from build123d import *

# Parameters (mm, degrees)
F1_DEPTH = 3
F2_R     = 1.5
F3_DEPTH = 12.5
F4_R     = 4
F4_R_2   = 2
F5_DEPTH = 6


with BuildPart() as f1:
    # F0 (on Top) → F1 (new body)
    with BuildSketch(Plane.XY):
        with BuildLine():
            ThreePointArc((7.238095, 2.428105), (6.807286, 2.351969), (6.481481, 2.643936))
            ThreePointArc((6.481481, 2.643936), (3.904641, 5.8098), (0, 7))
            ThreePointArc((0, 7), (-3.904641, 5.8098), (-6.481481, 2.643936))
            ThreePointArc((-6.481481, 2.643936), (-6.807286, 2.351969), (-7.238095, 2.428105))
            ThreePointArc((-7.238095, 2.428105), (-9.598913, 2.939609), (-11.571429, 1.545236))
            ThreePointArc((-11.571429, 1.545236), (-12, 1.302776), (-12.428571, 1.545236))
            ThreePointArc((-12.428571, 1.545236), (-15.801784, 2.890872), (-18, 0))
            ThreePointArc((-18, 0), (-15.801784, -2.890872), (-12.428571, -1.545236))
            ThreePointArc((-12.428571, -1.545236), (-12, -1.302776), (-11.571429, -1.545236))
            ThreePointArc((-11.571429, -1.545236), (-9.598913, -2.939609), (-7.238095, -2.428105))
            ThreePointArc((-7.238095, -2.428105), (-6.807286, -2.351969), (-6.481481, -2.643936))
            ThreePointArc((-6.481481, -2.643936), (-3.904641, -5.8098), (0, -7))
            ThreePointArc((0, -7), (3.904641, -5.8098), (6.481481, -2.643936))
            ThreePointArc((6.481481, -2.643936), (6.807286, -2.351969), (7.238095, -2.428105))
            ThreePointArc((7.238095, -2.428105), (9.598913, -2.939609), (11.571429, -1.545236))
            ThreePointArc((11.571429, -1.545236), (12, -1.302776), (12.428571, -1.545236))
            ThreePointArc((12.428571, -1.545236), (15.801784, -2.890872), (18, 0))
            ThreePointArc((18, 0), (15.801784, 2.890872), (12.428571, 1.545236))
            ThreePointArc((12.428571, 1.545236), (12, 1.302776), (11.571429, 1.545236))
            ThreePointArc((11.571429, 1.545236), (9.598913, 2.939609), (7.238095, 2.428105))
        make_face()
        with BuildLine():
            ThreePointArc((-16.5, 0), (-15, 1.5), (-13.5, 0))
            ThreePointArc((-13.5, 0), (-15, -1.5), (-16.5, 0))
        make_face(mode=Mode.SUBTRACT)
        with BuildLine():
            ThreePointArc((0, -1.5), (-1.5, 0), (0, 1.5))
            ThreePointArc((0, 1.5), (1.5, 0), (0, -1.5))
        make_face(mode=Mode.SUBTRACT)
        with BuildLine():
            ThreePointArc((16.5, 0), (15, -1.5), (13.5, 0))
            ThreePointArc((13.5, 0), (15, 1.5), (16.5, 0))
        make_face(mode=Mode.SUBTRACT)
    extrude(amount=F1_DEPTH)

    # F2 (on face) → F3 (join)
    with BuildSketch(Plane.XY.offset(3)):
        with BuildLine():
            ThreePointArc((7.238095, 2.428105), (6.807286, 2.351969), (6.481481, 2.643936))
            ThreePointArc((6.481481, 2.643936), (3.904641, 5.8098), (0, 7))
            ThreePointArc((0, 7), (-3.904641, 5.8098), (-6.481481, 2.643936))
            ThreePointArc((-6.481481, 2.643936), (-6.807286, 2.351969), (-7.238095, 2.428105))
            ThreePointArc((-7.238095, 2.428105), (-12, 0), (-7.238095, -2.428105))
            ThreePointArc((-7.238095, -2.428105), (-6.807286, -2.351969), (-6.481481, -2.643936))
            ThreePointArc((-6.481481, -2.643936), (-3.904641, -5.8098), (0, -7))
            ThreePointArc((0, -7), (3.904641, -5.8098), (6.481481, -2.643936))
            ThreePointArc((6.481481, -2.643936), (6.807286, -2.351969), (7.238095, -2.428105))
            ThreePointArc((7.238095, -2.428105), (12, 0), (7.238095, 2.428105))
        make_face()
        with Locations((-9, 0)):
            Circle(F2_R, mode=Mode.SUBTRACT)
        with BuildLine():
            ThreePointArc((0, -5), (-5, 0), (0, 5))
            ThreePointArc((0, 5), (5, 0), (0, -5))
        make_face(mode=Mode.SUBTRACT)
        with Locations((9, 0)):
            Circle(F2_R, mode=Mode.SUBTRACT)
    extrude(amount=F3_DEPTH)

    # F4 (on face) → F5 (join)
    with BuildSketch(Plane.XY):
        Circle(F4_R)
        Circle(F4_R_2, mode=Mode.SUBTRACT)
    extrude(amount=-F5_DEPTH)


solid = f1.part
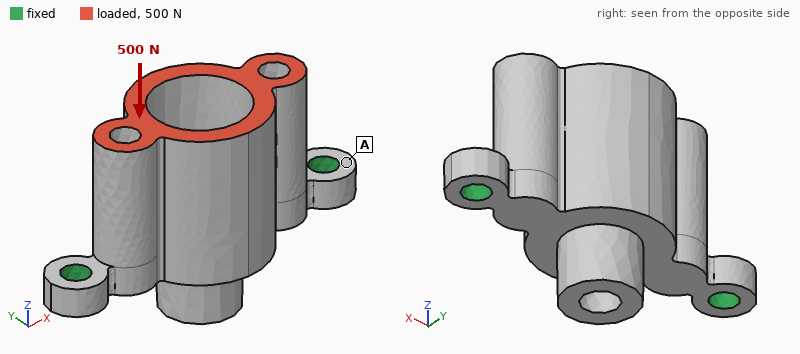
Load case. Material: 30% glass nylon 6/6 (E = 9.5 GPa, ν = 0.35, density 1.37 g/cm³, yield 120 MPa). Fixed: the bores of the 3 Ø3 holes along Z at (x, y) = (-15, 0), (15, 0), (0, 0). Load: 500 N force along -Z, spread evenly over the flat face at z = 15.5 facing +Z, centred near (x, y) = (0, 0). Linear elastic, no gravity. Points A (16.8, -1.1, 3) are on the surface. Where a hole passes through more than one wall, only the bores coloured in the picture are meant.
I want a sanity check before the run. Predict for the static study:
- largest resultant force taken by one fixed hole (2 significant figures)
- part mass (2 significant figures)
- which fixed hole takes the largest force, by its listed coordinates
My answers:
350 N
3.2 g
(0, 0)
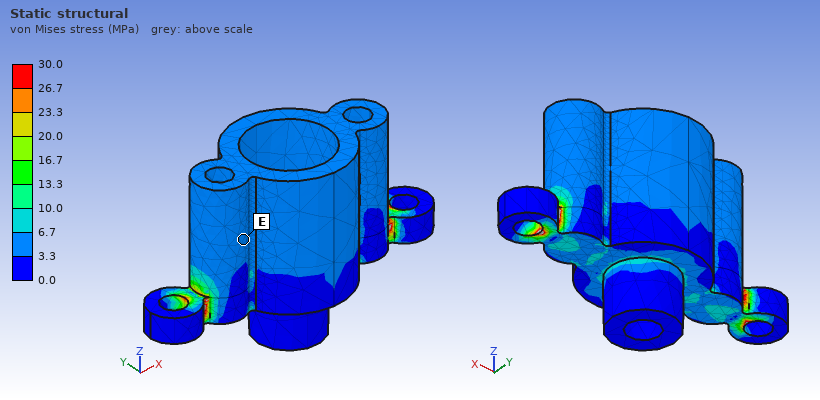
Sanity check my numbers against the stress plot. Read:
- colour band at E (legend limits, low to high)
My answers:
3.3 to 6.7 MPa
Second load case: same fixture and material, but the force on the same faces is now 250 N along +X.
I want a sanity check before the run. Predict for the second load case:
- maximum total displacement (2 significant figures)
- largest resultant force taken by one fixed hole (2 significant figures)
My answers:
49 µm
140 N
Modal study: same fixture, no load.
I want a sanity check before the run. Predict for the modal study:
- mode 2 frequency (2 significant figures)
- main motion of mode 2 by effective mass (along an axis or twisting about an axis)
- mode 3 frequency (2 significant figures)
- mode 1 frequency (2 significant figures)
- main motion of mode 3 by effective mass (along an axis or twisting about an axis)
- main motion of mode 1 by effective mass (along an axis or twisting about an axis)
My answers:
13 kHz
along X
14 kHz
5900 Hz
twisting about Z
along Y
